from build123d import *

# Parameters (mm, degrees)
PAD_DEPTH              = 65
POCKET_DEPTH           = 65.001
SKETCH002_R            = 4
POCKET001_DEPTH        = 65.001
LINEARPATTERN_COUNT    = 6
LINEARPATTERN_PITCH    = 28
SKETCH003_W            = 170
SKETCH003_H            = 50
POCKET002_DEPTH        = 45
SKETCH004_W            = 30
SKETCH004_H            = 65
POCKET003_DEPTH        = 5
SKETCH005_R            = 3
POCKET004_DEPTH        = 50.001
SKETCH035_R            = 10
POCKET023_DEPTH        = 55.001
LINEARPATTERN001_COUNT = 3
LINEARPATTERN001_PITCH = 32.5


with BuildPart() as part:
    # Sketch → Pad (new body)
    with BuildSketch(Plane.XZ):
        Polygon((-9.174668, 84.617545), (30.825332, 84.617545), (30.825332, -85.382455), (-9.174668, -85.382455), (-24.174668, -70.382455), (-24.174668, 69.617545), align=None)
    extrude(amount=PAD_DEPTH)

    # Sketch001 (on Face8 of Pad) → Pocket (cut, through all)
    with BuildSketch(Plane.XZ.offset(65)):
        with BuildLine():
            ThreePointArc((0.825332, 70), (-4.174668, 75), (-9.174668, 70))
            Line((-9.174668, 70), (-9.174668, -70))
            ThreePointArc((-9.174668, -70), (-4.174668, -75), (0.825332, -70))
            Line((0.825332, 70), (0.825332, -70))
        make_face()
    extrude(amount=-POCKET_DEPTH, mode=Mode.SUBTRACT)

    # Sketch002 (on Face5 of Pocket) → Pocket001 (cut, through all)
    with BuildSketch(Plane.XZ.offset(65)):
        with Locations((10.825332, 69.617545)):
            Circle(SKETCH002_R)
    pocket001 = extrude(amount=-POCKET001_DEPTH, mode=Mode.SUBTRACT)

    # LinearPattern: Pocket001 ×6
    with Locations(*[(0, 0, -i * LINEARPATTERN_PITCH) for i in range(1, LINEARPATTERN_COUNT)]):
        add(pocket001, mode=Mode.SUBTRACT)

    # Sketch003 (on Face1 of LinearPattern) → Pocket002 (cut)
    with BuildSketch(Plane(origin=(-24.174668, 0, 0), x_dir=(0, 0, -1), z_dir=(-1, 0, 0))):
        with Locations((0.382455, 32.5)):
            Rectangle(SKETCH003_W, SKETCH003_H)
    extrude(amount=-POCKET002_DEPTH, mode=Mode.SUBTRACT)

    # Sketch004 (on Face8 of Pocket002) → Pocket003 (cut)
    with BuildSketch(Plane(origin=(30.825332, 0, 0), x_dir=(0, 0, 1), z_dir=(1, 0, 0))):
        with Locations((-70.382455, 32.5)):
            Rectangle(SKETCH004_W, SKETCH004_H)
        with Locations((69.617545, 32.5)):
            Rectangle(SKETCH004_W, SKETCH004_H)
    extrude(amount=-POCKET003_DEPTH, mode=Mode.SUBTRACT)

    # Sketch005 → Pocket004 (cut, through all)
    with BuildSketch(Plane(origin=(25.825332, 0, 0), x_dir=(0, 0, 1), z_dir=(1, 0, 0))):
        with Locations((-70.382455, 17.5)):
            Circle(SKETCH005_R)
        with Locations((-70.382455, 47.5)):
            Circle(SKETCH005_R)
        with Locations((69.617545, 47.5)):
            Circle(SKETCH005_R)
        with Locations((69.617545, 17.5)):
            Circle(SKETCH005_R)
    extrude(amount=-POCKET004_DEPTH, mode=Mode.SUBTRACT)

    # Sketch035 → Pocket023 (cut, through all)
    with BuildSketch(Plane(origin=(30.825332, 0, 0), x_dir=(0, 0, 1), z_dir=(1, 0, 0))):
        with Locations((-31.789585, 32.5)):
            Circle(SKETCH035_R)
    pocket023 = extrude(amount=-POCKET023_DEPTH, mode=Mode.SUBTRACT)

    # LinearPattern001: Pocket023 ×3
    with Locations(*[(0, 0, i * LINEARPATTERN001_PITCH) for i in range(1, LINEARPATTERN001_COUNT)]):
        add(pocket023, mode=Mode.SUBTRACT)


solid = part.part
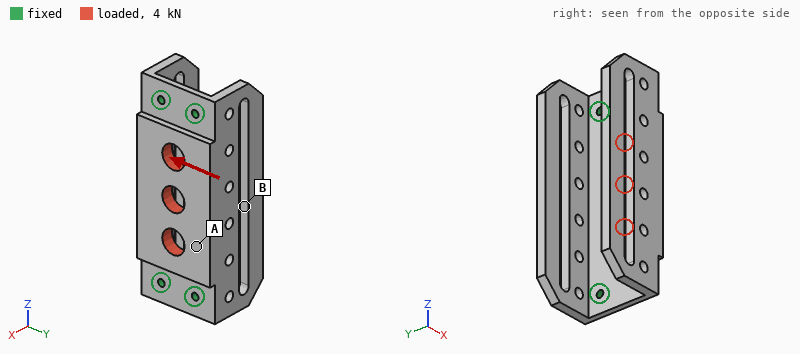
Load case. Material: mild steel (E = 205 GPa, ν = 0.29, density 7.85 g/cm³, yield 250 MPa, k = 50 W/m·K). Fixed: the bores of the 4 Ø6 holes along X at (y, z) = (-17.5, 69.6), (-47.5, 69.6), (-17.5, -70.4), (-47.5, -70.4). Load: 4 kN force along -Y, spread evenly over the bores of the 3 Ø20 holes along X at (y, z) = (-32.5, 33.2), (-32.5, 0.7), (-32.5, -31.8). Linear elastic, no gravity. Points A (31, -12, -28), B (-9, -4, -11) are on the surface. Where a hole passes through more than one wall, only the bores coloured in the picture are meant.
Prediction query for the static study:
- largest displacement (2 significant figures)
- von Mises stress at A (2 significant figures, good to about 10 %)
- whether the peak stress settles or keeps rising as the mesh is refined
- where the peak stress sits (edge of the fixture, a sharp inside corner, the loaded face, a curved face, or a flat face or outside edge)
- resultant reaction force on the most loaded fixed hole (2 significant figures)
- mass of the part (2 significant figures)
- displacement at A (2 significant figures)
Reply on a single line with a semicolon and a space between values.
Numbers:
6.5 µm; 5.9 MPa; keeps rising; edge of the fixture; 1.2 kN; 1.3 kg; 4.4 µm
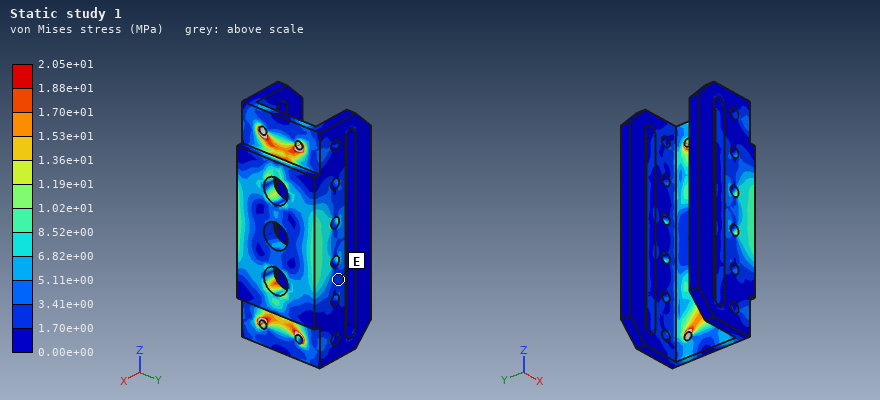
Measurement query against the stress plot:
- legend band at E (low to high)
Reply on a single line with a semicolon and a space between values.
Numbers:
1.70e+00 to 3.41e+00 MPa
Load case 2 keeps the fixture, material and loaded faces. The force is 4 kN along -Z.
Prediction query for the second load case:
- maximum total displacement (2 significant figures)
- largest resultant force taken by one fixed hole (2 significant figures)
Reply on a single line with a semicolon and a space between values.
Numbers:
1.8 µm; 1.0 kN
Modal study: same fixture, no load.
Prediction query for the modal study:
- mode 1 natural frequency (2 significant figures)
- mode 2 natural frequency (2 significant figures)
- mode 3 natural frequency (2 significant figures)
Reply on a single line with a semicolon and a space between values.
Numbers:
820 Hz; 840 Hz; 1900 Hz
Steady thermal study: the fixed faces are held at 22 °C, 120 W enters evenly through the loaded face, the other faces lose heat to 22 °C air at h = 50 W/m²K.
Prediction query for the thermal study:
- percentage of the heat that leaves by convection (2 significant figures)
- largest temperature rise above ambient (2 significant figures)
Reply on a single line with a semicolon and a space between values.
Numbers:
55 %; 72 K
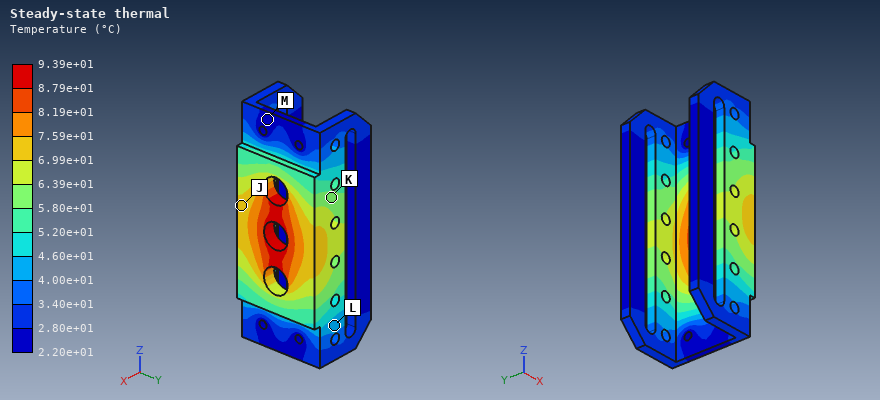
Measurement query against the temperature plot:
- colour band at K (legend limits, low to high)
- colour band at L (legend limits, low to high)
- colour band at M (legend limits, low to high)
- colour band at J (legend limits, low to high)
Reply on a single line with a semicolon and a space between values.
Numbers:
5.80e+01 to 6.39e+01 °C; 4.00e+01 to 4.60e+01 °C; 2.20e+01 to 2.80e+01 °C; 6.99e+01 to 7.59e+01 °C
